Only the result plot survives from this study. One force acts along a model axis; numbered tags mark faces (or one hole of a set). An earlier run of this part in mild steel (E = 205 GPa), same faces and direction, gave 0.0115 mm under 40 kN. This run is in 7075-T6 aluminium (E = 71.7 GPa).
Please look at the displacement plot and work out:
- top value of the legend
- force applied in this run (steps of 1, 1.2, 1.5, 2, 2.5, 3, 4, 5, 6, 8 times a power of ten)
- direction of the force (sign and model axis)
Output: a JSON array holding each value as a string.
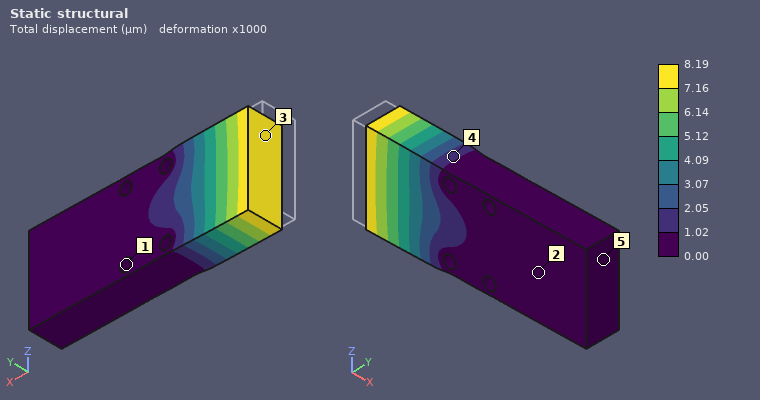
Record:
["8.19 µm", "10 kN", "+X"]
